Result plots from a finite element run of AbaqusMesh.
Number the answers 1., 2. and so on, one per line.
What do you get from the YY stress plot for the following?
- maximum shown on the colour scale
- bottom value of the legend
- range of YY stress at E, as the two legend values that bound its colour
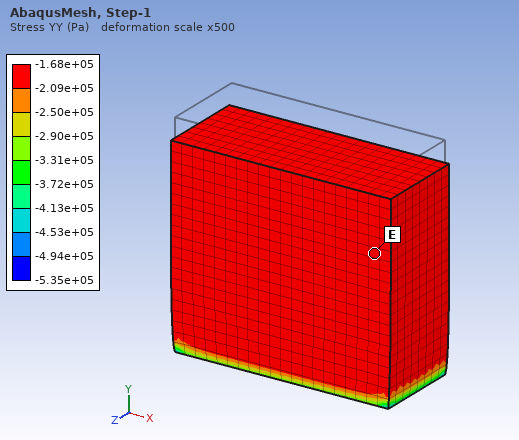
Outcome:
1. -1.68e+05 Pa
2. -5.35e+05 Pa
3. -2.09e+05 to -1.68e+05 Pa
